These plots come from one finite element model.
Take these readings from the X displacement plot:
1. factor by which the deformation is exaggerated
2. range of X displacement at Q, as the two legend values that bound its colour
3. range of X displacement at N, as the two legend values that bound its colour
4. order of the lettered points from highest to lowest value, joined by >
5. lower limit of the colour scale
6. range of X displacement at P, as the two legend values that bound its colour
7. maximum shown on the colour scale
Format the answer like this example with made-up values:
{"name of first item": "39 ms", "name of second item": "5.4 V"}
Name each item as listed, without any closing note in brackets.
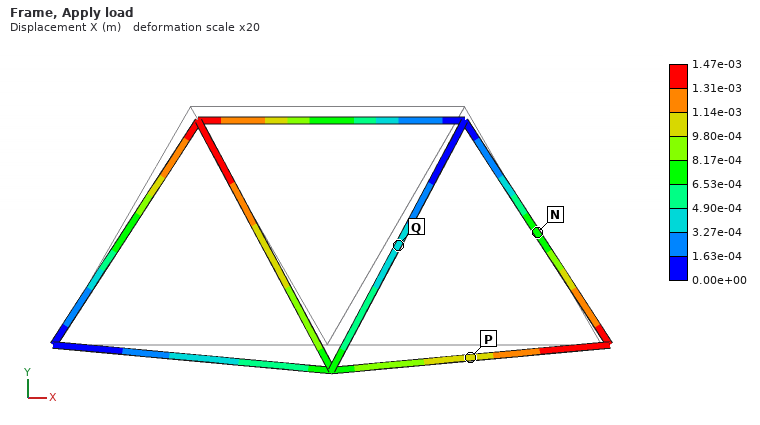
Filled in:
{"factor by which the deformation is exaggerated": "20", "range of X displacement at Q, as the two legend values that bound its colour": "3.27e-04 to 4.90e-04 m", "range of X displacement at N, as the two legend values that bound its colour": "6.53e-04 to 8.17e-04 m", "order of the lettered points from highest to lowest value, joined by >": "P > N > Q", "lower limit of the colour scale": "0.00e+00 m", "range of X displacement at P, as the two legend values that bound its colour": "9.80e-04 to 1.14e-03 m", "maximum shown on the colour scale": "1.47e-03 m"}
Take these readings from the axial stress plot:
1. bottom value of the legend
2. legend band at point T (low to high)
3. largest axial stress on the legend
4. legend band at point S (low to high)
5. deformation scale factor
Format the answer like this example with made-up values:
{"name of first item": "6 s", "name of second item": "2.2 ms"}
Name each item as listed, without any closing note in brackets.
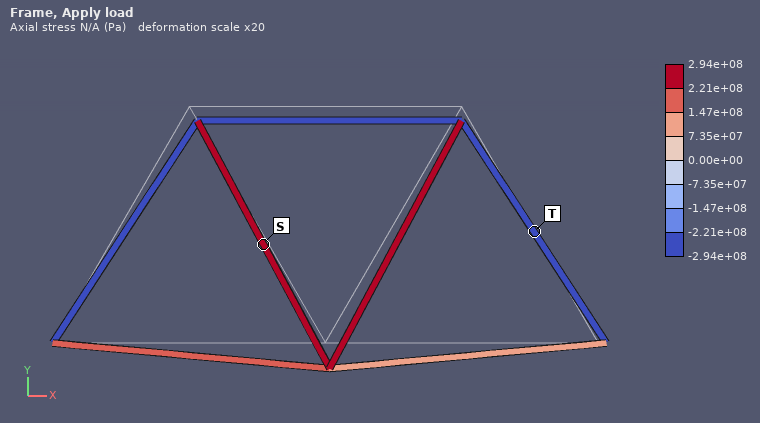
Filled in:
{"bottom value of the legend": "-2.94e+08 Pa", "legend band at point T": "-2.94e+08 to -2.21e+08 Pa", "largest axial stress on the legend": "2.94e+08 Pa", "legend band at point S": "2.21e+08 to 2.94e+08 Pa", "deformation scale factor": "20"}
